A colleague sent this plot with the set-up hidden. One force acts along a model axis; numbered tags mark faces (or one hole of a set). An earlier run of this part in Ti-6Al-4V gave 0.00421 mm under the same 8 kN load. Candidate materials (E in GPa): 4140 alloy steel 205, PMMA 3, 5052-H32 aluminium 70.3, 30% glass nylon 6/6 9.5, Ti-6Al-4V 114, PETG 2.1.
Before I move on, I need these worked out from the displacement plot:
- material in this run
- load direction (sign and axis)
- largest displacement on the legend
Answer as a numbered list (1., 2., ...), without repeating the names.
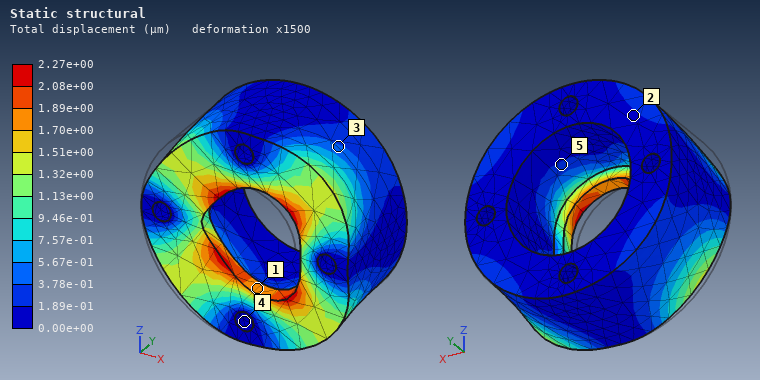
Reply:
1. 4140 alloy steel
2. +X
3. 2.27e+00 µm
